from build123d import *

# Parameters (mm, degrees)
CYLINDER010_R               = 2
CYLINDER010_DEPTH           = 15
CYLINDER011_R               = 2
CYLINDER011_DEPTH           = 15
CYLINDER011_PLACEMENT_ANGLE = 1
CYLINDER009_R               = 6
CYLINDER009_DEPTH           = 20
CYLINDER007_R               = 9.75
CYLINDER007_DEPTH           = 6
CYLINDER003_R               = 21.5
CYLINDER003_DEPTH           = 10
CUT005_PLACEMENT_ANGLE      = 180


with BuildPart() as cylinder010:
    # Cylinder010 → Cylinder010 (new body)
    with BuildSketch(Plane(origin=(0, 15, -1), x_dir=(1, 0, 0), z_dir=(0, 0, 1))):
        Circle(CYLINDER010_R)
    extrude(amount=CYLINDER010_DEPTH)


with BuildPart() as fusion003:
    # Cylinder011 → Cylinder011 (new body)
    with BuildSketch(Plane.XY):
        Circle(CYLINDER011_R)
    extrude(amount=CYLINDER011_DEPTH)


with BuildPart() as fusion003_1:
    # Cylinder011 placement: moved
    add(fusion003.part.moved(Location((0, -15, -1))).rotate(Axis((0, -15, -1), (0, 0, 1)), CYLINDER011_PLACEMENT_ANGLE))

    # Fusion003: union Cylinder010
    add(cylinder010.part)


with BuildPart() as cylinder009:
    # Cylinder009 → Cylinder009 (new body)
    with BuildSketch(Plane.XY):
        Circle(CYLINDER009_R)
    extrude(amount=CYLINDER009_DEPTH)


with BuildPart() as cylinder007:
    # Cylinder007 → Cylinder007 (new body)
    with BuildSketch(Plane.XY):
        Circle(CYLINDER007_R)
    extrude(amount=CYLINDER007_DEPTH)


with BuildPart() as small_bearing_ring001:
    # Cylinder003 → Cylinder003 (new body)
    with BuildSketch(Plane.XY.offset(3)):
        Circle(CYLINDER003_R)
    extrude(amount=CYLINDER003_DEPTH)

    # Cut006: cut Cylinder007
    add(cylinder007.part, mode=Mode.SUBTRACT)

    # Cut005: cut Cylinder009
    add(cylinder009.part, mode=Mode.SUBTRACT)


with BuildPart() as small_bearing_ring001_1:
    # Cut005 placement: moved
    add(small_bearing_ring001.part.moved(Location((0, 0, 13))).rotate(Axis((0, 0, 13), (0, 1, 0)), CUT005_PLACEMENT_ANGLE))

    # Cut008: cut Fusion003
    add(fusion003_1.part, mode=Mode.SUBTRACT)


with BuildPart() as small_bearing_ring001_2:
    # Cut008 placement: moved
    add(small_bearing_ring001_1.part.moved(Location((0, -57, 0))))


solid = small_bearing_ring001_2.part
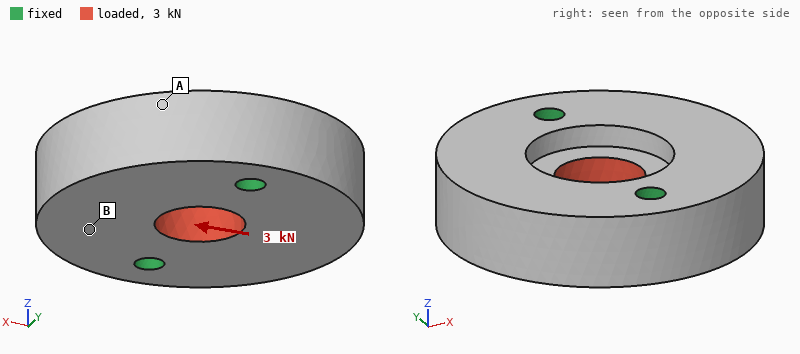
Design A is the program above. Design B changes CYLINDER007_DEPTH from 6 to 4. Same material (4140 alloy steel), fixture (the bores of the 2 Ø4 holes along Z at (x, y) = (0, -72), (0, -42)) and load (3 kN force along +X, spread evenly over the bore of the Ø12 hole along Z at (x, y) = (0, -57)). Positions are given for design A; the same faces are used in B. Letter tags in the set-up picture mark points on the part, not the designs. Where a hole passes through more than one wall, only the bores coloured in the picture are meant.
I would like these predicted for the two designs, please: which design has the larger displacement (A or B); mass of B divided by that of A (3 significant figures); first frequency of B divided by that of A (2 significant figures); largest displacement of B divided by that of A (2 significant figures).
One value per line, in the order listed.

A
1.03
1.0
0.78
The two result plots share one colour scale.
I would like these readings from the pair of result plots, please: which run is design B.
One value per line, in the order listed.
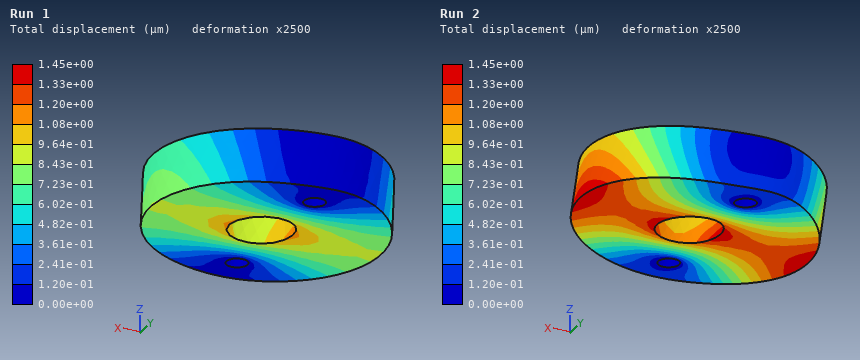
Run 1
